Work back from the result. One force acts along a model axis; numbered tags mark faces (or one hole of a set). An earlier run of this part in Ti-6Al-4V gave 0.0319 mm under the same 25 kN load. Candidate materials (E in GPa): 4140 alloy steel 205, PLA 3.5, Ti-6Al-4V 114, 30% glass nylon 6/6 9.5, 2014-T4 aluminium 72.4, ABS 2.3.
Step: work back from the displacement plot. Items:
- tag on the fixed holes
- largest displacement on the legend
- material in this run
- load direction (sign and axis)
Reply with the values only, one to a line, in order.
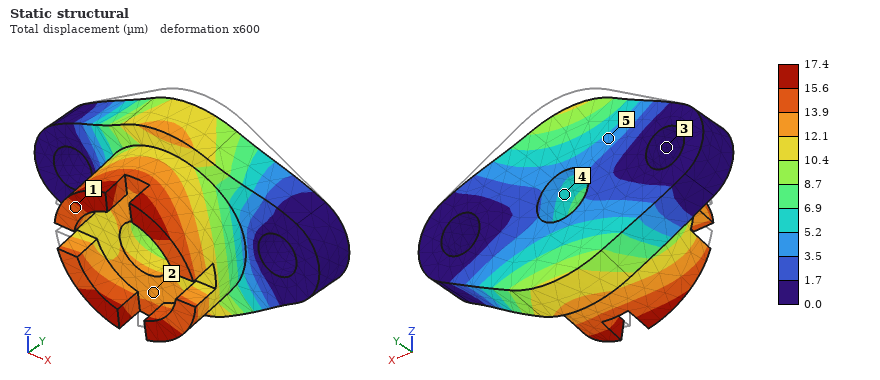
3
17.4 µm
4140 alloy steel
-Z
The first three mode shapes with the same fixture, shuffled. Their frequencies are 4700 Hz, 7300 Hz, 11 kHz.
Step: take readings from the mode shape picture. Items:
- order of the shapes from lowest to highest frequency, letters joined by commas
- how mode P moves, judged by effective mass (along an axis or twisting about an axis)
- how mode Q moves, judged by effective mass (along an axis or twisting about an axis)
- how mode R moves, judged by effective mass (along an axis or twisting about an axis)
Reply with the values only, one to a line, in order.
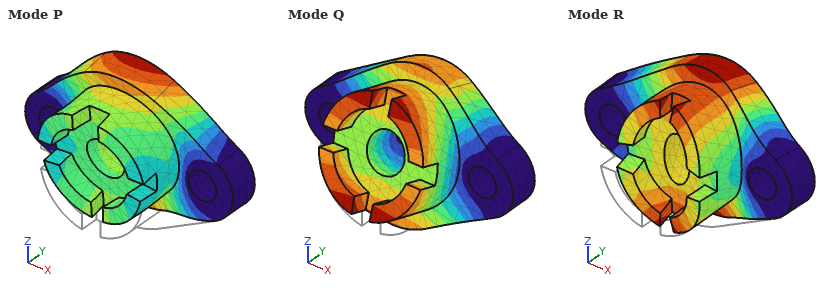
Q, R, P
along Z
along Z
along Y
